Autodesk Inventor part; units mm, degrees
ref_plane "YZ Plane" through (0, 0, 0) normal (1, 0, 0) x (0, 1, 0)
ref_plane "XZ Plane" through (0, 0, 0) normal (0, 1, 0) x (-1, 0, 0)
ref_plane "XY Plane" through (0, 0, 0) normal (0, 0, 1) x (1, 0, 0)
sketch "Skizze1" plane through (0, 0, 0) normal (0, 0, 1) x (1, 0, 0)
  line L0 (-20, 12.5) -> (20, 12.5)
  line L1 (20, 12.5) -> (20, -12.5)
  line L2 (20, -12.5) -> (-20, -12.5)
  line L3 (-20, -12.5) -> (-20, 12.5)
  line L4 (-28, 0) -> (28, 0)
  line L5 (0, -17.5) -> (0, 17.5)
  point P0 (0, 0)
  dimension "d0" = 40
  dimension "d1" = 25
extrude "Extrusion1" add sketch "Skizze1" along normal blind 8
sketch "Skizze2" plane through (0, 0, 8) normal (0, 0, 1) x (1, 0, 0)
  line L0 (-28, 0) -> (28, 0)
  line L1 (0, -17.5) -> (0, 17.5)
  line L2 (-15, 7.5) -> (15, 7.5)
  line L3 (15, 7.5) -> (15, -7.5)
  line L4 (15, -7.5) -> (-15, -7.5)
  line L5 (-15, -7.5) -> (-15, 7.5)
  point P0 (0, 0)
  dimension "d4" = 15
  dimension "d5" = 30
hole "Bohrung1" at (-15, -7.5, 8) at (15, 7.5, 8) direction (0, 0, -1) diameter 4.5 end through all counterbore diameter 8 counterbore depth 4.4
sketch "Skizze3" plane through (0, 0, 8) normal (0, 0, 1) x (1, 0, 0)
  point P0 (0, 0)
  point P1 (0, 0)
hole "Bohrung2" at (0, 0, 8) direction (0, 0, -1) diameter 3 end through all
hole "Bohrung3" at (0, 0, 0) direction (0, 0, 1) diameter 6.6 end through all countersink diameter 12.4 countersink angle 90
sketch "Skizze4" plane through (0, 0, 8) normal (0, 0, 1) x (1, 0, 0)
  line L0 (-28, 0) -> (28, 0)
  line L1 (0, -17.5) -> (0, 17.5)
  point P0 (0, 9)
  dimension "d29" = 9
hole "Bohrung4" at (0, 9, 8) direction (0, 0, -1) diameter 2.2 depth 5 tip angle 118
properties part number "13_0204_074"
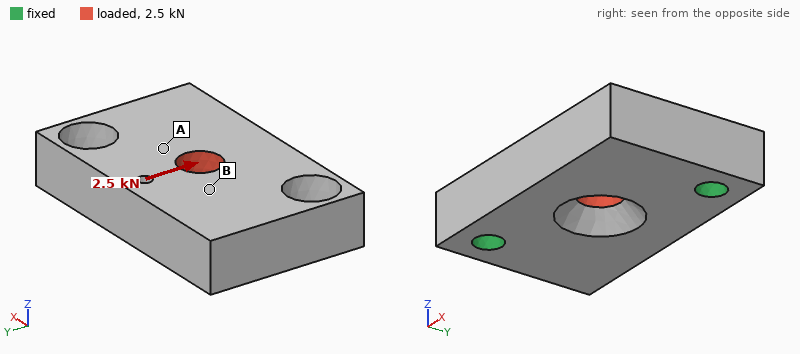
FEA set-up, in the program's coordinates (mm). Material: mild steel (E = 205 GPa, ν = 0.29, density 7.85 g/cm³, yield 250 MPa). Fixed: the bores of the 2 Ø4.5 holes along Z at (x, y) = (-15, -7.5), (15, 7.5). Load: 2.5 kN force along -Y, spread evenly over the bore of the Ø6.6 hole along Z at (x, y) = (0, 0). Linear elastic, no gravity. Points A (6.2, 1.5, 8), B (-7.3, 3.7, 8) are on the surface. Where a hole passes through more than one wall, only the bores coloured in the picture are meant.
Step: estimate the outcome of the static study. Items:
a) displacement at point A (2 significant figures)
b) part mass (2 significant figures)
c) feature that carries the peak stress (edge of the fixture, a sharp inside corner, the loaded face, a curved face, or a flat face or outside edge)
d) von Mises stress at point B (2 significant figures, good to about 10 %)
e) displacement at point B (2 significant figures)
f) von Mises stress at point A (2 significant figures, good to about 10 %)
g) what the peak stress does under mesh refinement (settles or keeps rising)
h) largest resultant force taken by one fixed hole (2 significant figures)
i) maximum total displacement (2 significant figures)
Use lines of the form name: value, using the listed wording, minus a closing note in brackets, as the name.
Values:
displacement at point A: 5.1 µm
part mass: 55 g
feature that carries the peak stress: edge of the fixture
von Mises stress at point B: 12 MPa
displacement at point B: 6.2 µm
von Mises stress at point A: 22 MPa
what the peak stress does under mesh refinement: keeps rising
largest resultant force taken by one fixed hole: 1.3 kN
maximum total displacement: 11 µm
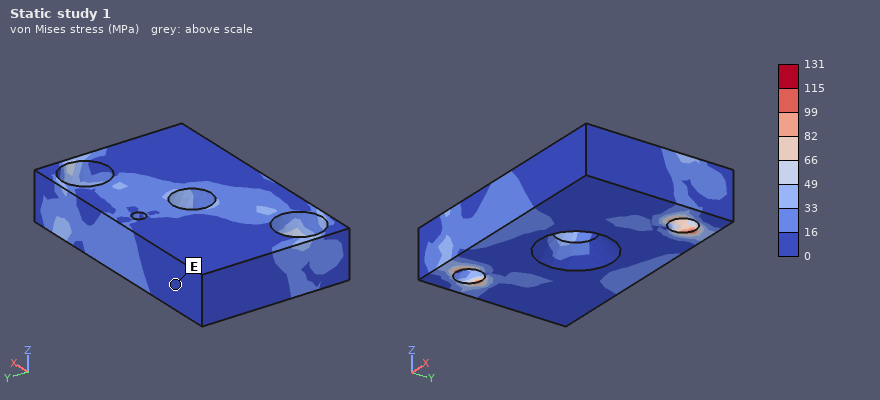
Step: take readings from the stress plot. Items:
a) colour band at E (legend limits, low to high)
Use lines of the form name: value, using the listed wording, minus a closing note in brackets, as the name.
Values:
colour band at E: 0 to 16 MPa
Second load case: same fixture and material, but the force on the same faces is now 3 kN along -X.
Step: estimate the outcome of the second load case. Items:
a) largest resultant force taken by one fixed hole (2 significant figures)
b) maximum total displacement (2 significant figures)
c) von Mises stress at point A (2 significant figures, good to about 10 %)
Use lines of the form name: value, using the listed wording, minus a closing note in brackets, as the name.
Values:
largest resultant force taken by one fixed hole: 1.5 kN
maximum total displacement: 7.3 µm
von Mises stress at point A: 29 MPa
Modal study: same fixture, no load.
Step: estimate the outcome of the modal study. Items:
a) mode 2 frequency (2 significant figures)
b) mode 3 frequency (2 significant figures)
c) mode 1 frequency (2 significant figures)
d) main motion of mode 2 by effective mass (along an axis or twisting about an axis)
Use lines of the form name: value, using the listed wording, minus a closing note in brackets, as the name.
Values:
mode 2 frequency: 15 kHz
mode 3 frequency: 26 kHz
mode 1 frequency: 9000 Hz
main motion of mode 2 by effective mass: along Z
